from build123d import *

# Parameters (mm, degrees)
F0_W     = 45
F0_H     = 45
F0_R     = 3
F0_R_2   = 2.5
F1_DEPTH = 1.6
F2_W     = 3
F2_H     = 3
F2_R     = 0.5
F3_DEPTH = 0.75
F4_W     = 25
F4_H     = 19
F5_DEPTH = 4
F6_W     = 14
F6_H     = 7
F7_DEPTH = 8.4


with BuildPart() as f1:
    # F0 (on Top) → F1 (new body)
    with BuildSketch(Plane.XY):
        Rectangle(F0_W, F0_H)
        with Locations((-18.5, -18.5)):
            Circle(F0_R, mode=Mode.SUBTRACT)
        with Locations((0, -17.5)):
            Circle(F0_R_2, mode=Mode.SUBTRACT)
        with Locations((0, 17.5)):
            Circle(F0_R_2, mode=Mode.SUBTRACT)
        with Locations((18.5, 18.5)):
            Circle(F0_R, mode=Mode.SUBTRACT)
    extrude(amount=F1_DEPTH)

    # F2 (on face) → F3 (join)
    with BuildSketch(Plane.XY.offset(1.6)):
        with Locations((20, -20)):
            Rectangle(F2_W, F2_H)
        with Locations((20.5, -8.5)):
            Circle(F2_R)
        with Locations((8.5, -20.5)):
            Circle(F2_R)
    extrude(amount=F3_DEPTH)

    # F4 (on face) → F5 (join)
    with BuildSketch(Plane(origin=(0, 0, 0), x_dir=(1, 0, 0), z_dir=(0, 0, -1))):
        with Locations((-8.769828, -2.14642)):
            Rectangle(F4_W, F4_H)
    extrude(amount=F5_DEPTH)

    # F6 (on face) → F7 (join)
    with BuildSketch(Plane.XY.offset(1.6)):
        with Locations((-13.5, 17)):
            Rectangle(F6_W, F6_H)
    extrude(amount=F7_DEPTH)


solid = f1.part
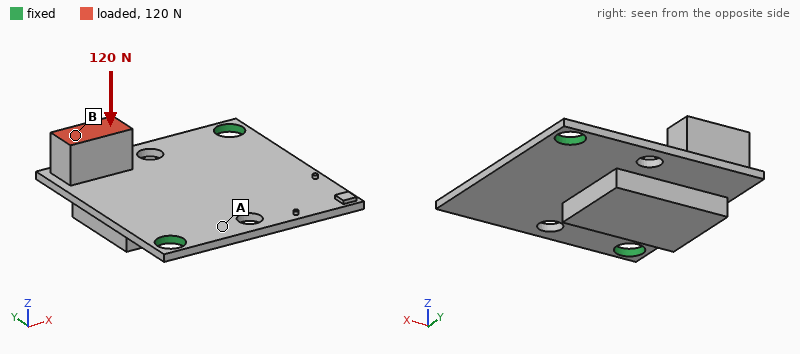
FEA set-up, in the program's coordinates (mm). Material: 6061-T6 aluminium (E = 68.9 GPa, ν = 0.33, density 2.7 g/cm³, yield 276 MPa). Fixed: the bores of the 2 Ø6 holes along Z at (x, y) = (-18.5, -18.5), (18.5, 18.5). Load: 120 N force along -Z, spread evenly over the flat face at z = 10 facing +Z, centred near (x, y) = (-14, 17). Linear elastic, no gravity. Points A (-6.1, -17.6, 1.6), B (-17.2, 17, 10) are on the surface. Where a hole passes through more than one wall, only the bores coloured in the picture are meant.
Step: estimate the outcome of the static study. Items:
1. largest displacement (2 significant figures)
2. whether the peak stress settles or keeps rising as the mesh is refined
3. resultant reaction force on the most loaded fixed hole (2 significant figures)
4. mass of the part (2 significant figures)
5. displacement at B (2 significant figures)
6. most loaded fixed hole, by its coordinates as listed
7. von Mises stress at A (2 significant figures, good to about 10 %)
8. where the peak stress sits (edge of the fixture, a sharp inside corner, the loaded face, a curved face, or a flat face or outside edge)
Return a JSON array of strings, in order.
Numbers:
["0.55 mm", "keeps rising", "120 N", "16 g", "0.45 mm", "(18.5, 18.5)", "36 MPa", "edge of the fixture"]
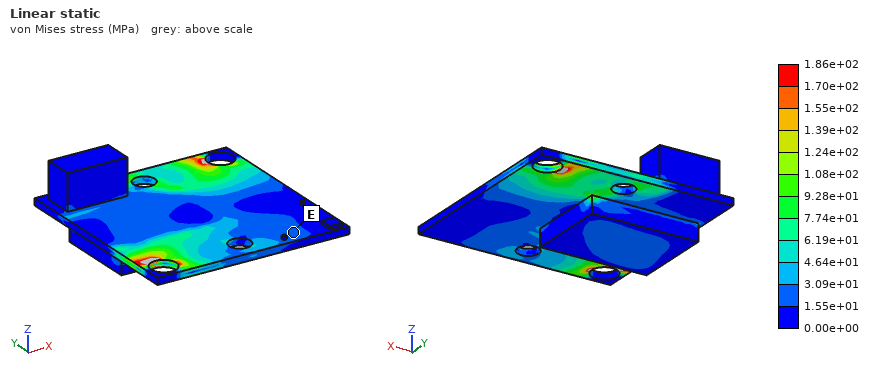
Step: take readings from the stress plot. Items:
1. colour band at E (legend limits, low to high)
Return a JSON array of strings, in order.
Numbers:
["1.55e+01 to 3.09e+01 MPa"]
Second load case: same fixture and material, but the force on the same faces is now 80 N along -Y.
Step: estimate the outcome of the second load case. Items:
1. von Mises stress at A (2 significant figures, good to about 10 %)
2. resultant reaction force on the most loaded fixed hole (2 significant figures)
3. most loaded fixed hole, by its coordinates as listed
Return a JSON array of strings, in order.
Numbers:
["7.7 MPa", "65 N", "(-18.5, -18.5)"]
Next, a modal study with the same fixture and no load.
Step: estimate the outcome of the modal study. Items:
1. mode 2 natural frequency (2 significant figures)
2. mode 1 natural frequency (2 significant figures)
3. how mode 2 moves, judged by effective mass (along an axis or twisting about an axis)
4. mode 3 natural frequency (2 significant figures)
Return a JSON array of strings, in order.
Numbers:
["2300 Hz", "1200 Hz", "along Z", "4700 Hz"]
